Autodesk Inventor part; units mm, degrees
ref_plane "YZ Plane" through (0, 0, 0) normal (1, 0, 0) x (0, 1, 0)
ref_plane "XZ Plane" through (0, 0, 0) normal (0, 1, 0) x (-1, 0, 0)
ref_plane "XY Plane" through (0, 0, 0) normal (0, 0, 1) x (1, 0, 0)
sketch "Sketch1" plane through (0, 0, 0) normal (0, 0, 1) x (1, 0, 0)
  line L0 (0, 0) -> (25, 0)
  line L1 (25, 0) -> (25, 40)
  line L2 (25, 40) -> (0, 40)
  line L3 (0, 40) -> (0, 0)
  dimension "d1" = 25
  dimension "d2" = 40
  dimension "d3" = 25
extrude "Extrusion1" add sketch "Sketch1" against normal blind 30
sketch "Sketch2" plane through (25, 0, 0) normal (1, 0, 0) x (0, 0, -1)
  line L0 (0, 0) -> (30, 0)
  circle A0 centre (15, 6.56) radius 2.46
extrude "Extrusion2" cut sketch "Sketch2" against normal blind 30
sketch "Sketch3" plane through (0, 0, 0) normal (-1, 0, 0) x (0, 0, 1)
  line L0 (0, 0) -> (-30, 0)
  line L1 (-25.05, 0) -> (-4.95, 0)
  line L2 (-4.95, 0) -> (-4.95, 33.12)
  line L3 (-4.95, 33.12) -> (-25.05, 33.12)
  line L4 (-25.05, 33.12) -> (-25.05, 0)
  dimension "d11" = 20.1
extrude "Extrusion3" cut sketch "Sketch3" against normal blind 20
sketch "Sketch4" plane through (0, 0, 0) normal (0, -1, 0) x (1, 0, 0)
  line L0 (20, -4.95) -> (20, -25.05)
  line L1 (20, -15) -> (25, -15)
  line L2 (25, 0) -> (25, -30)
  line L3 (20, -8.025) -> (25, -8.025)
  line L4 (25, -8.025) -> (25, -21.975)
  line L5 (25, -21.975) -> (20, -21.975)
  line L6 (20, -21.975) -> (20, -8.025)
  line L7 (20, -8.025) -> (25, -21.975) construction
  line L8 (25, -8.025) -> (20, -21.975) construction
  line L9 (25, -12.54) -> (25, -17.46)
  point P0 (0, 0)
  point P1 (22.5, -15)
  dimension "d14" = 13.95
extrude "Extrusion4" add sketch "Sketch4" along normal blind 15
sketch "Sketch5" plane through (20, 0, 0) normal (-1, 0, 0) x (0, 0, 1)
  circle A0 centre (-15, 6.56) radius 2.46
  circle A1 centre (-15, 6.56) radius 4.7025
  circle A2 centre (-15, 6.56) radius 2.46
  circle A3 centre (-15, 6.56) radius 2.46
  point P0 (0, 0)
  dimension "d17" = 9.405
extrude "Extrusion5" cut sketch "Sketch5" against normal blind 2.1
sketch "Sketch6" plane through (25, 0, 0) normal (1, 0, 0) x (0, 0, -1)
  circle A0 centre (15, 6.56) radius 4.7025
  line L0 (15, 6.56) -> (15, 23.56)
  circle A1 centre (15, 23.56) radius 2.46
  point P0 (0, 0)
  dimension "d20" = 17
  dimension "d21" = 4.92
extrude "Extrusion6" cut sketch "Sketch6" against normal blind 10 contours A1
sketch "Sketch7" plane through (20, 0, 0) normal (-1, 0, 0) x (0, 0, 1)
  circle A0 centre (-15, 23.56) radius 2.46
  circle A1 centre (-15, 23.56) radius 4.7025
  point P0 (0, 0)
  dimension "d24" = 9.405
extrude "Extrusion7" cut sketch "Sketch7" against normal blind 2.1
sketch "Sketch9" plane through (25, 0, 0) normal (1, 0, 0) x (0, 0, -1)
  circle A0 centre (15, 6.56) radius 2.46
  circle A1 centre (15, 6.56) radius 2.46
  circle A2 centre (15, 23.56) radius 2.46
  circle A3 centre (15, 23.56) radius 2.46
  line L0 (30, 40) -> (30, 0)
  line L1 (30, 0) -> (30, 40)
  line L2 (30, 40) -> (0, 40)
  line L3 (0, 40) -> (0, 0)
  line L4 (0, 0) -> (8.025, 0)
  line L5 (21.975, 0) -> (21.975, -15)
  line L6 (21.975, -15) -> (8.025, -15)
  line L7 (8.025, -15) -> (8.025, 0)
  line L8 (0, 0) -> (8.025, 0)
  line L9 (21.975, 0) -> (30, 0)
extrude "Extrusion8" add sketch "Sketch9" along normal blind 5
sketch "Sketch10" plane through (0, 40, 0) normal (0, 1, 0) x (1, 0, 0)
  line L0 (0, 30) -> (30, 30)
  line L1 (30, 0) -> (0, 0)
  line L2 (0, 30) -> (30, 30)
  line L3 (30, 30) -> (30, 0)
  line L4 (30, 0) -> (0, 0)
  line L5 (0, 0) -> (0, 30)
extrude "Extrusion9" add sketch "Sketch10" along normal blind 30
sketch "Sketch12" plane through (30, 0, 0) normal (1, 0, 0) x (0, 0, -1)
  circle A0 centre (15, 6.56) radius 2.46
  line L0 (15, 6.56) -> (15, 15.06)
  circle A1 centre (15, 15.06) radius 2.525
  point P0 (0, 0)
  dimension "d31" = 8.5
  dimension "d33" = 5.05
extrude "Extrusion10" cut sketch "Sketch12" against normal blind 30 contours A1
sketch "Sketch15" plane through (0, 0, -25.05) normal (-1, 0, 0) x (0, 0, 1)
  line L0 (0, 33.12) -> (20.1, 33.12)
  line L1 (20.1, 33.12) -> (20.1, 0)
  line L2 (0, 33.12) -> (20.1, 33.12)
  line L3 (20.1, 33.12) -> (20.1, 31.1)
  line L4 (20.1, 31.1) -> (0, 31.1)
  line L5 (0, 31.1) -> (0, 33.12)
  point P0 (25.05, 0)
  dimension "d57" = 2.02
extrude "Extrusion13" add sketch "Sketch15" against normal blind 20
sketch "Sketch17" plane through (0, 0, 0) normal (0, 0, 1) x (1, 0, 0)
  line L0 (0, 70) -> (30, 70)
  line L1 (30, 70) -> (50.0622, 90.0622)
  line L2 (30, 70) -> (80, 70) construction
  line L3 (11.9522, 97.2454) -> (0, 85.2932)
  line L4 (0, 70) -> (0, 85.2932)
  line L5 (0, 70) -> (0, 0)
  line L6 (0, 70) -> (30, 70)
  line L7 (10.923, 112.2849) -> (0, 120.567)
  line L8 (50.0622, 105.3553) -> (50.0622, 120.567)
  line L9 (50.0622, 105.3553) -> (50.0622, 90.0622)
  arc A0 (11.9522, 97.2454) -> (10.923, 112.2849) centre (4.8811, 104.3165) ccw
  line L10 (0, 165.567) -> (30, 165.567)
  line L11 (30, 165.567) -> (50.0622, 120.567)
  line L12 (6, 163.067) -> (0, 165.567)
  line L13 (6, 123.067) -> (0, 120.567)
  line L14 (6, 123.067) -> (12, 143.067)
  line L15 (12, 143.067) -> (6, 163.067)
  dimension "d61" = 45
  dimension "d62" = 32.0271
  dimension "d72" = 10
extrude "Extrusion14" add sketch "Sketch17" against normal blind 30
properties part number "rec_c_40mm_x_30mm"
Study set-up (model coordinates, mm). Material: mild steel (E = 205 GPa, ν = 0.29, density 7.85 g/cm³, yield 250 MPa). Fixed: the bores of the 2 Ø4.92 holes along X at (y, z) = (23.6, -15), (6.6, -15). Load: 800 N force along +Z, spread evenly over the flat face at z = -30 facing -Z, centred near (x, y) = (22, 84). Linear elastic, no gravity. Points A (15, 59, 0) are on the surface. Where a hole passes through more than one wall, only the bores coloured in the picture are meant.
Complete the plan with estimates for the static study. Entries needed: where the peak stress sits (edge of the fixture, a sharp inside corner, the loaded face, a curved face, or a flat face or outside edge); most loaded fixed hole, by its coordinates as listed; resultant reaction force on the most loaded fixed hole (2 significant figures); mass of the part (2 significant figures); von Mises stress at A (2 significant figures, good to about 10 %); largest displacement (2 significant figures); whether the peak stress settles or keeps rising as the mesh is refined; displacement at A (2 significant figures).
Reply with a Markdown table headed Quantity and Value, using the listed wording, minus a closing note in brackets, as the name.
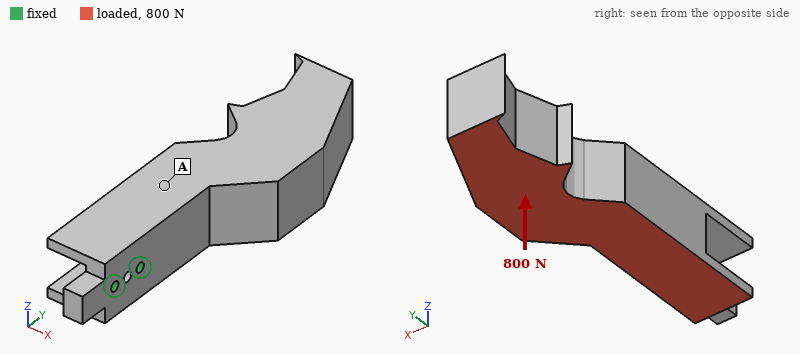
| Quantity | Value |
|---|---|
| where the peak stress sits | edge of the fixture |
| most loaded fixed hole, by its coordinates as listed | (23.6, -15) |
| resultant reaction force on the most loaded fixed hole | 2.9 kN |
| mass of the part | 1.2 kg |
| von Mises stress at A | 6.1 MPa |
| largest displacement | 52 µm |
| whether the peak stress settles or keeps rising as the mesh is refined | keeps rising |
| displacement at A | 11 µm |
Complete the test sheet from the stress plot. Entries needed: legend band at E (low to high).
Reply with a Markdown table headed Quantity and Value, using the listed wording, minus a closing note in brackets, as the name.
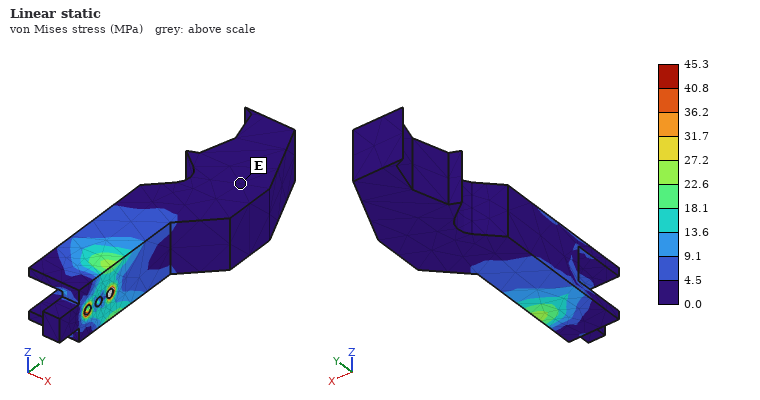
| Quantity | Value |
|---|---|
| legend band at E | 0.0 to 4.5 MPa |
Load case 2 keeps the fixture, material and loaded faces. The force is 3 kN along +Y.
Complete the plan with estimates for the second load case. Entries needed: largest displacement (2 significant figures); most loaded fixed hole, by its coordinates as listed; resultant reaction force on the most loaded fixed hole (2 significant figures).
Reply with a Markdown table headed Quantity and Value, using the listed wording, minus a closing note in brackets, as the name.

| Quantity | Value |
|---|---|
| largest displacement | 50 µm |
| most loaded fixed hole, by its coordinates as listed | (23.6, -15) |
| resultant reaction force on the most loaded fixed hole | 2.9 kN |
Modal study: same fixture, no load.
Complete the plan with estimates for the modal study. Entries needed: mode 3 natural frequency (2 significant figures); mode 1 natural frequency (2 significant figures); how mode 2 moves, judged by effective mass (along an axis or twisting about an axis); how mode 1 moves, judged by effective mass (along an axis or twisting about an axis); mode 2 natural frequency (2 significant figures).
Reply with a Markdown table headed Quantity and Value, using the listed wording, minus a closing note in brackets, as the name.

| Quantity | Value |
|---|---|
| mode 3 natural frequency | 2300 Hz |
| mode 1 natural frequency | 590 Hz |
| how mode 2 moves, judged by effective mass | along Z |
| how mode 1 moves, judged by effective mass | along X |
| mode 2 natural frequency | 680 Hz |
